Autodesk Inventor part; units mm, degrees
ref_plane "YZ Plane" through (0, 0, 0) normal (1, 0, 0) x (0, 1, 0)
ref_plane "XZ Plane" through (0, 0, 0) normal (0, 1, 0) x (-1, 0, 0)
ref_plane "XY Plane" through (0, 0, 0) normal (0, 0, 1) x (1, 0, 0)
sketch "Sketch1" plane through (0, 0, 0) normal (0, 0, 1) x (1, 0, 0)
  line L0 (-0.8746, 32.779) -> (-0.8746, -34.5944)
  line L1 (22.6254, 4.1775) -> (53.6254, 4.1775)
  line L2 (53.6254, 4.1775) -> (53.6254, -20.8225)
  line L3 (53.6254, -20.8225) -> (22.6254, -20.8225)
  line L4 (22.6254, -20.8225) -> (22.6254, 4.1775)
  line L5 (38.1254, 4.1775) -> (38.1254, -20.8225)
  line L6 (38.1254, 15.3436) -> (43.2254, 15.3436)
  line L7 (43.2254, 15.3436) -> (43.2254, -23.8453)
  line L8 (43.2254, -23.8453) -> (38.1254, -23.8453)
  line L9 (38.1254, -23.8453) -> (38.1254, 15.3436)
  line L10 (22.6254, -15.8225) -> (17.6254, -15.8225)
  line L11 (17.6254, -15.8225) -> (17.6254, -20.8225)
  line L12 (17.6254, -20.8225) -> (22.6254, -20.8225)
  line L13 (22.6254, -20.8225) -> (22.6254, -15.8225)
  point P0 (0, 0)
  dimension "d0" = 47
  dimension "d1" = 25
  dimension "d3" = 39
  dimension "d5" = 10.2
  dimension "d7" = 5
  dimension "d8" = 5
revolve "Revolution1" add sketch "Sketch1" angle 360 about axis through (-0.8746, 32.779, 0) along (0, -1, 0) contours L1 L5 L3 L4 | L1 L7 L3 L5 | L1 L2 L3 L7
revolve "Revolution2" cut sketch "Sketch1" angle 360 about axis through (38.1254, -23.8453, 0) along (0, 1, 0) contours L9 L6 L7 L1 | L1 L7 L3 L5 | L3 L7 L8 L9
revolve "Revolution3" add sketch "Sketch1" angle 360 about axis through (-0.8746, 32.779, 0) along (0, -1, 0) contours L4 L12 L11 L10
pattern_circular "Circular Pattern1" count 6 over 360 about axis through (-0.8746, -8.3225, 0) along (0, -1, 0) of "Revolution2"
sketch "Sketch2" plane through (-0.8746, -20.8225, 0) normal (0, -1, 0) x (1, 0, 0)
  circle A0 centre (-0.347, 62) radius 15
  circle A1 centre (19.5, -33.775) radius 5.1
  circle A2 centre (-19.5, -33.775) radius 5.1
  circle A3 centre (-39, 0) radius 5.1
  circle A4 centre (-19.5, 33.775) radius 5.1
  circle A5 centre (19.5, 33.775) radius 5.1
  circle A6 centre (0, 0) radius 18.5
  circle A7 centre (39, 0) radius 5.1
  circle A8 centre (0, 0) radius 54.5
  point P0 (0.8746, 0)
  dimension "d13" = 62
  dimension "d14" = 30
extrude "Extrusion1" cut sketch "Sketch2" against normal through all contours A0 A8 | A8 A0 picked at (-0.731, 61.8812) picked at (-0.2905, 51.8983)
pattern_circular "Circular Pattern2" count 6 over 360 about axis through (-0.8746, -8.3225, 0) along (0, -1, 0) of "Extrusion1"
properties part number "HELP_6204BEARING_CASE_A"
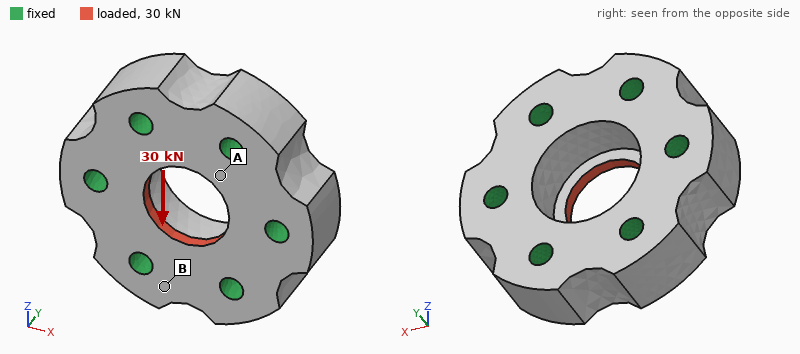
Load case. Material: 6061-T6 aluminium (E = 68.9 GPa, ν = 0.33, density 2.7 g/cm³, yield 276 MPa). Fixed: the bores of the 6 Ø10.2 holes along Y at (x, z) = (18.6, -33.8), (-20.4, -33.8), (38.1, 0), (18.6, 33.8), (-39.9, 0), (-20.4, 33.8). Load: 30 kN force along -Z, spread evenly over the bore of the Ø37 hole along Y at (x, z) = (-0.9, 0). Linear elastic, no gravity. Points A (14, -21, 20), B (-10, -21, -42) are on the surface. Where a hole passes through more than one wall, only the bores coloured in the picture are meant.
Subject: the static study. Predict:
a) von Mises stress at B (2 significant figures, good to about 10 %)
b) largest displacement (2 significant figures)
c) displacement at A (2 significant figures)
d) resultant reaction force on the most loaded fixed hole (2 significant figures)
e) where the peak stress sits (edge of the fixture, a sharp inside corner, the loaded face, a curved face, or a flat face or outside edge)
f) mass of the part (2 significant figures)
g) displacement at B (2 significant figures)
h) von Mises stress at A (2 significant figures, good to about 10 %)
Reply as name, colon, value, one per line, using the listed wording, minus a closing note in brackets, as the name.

von Mises stress at B: 13 MPa
largest displacement: 17 µm
displacement at A: 8.2 µm
resultant reaction force on the most loaded fixed hole: 6.6 kN
where the peak stress sits: a sharp inside corner
mass of the part: 440 g
displacement at B: 2.7 µm
von Mises stress at A: 52 MPa
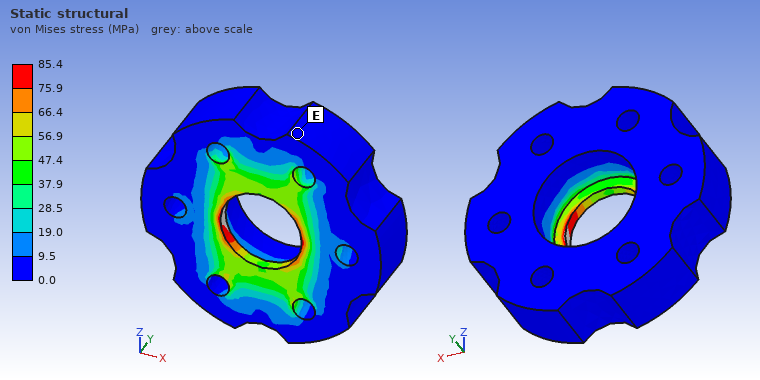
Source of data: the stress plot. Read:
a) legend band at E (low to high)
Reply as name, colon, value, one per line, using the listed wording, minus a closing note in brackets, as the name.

legend band at E: 0.0 to 9.5 MPa
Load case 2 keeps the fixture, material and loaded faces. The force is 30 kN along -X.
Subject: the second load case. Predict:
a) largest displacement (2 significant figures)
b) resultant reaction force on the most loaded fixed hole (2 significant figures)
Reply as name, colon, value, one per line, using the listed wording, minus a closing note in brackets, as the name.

largest displacement: 16 µm
resultant reaction force on the most loaded fixed hole: 7.5 kN
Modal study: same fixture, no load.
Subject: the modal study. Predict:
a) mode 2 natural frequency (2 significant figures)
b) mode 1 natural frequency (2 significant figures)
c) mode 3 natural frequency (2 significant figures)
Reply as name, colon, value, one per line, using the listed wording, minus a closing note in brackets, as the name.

mode 2 natural frequency: 36 kHz
mode 1 natural frequency: 34 kHz
mode 3 natural frequency: 36 kHz
